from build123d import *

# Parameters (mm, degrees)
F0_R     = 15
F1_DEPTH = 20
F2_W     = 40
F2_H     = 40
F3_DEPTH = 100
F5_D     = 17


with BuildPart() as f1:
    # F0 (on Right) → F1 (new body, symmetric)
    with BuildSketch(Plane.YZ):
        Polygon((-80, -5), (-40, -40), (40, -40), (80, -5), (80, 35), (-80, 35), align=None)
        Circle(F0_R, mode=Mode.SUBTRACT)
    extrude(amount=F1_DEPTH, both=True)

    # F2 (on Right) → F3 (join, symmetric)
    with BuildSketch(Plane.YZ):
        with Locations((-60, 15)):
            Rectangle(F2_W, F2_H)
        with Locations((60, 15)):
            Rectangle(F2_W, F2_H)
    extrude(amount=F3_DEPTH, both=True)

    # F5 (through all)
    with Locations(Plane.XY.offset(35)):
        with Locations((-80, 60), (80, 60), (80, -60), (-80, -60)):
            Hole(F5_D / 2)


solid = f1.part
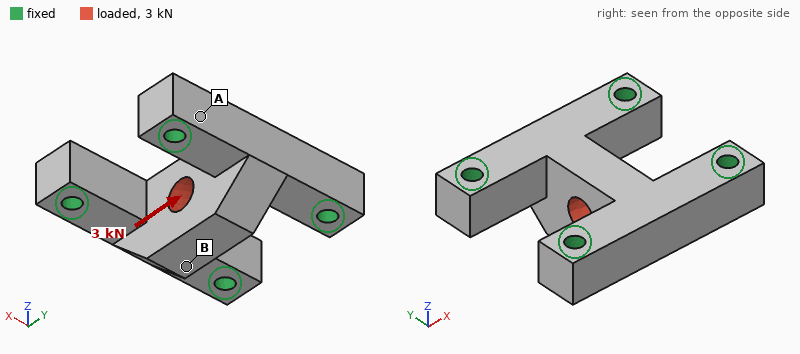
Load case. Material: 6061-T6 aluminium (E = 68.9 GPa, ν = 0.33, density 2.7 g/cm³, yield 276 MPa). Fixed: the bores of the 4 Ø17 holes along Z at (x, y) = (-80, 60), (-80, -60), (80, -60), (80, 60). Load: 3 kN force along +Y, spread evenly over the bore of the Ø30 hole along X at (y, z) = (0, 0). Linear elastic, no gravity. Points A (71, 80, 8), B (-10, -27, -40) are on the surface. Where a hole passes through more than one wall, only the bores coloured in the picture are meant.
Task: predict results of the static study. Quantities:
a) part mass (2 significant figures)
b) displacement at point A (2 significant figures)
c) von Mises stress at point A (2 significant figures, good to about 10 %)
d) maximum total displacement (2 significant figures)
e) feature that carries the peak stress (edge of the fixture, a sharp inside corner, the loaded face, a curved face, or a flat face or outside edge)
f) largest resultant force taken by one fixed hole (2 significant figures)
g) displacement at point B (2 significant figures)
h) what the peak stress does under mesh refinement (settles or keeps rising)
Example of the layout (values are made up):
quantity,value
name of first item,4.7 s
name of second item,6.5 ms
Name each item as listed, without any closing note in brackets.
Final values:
quantity,value
part mass,2.4 kg
displacement at point A,0.64 µm
von Mises stress at point A,1.4 MPa
maximum total displacement,4.1 µm
feature that carries the peak stress,edge of the fixture
largest resultant force taken by one fixed hole,780 N
displacement at point B,4.0 µm
what the peak stress does under mesh refinement,keeps rising
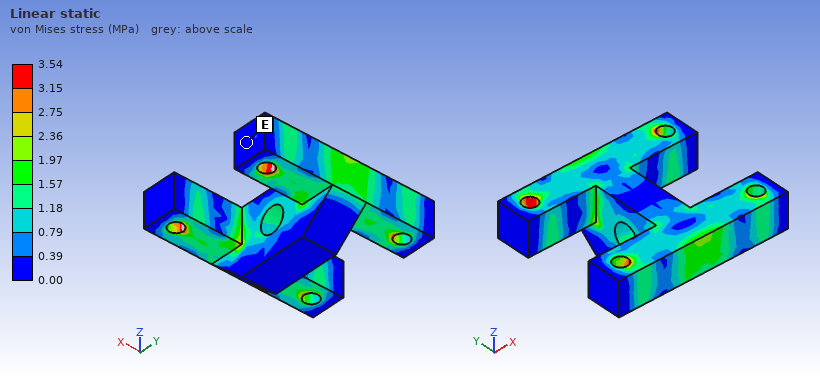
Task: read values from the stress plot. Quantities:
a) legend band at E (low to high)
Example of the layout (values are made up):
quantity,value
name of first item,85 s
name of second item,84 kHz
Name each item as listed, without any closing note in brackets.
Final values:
quantity,value
legend band at E,0.00 to 0.39 MPa
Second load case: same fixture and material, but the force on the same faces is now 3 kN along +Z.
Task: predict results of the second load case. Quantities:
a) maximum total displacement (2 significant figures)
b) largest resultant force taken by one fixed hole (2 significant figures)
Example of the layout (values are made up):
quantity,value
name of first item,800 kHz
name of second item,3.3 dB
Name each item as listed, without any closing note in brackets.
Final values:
quantity,value
maximum total displacement,4.7 µm
largest resultant force taken by one fixed hole,760 N
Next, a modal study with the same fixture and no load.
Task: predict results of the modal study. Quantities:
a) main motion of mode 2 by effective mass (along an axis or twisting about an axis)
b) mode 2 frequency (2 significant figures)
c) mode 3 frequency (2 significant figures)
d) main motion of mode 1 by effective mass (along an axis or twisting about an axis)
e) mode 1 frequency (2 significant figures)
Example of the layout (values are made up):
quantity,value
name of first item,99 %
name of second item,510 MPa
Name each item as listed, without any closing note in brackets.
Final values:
quantity,value
main motion of mode 2 by effective mass,along Z
mode 2 frequency,4500 Hz
mode 3 frequency,5800 Hz
main motion of mode 1 by effective mass,along Y
mode 1 frequency,4100 Hz
